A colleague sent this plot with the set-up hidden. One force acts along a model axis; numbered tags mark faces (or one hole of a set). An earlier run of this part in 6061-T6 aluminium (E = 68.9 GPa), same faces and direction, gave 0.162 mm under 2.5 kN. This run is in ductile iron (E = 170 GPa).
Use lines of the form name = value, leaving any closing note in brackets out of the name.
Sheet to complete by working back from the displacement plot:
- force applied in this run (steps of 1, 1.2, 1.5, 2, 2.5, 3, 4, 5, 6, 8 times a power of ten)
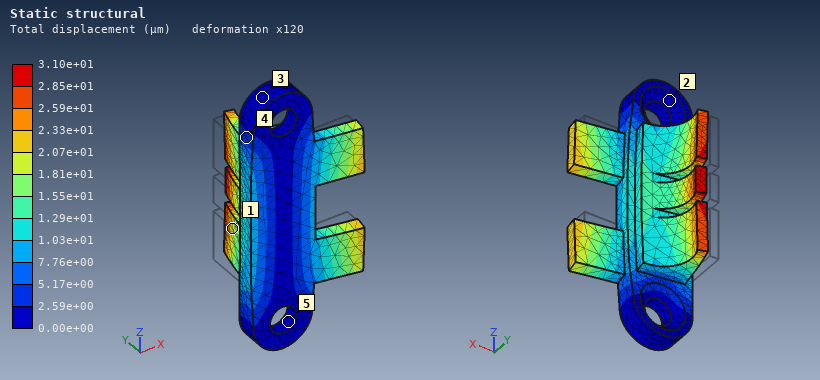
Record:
force applied in this run = 1.2 kN
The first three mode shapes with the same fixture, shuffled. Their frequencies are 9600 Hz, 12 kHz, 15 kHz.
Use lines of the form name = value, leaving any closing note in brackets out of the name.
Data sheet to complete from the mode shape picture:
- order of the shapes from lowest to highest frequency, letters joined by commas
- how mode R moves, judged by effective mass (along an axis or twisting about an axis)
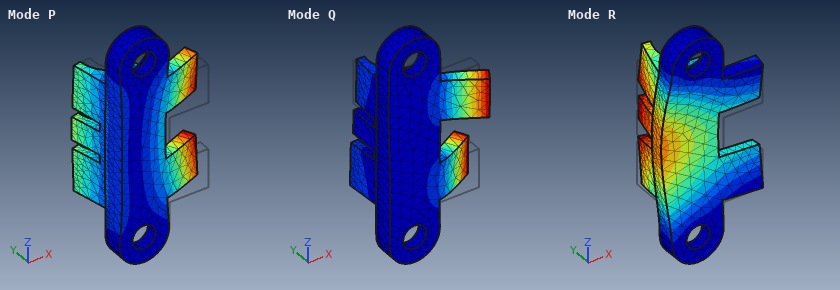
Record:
order of the shapes from lowest to highest frequency, letters joined by commas = P, R, Q
how mode R moves, judged by effective mass = along Y
